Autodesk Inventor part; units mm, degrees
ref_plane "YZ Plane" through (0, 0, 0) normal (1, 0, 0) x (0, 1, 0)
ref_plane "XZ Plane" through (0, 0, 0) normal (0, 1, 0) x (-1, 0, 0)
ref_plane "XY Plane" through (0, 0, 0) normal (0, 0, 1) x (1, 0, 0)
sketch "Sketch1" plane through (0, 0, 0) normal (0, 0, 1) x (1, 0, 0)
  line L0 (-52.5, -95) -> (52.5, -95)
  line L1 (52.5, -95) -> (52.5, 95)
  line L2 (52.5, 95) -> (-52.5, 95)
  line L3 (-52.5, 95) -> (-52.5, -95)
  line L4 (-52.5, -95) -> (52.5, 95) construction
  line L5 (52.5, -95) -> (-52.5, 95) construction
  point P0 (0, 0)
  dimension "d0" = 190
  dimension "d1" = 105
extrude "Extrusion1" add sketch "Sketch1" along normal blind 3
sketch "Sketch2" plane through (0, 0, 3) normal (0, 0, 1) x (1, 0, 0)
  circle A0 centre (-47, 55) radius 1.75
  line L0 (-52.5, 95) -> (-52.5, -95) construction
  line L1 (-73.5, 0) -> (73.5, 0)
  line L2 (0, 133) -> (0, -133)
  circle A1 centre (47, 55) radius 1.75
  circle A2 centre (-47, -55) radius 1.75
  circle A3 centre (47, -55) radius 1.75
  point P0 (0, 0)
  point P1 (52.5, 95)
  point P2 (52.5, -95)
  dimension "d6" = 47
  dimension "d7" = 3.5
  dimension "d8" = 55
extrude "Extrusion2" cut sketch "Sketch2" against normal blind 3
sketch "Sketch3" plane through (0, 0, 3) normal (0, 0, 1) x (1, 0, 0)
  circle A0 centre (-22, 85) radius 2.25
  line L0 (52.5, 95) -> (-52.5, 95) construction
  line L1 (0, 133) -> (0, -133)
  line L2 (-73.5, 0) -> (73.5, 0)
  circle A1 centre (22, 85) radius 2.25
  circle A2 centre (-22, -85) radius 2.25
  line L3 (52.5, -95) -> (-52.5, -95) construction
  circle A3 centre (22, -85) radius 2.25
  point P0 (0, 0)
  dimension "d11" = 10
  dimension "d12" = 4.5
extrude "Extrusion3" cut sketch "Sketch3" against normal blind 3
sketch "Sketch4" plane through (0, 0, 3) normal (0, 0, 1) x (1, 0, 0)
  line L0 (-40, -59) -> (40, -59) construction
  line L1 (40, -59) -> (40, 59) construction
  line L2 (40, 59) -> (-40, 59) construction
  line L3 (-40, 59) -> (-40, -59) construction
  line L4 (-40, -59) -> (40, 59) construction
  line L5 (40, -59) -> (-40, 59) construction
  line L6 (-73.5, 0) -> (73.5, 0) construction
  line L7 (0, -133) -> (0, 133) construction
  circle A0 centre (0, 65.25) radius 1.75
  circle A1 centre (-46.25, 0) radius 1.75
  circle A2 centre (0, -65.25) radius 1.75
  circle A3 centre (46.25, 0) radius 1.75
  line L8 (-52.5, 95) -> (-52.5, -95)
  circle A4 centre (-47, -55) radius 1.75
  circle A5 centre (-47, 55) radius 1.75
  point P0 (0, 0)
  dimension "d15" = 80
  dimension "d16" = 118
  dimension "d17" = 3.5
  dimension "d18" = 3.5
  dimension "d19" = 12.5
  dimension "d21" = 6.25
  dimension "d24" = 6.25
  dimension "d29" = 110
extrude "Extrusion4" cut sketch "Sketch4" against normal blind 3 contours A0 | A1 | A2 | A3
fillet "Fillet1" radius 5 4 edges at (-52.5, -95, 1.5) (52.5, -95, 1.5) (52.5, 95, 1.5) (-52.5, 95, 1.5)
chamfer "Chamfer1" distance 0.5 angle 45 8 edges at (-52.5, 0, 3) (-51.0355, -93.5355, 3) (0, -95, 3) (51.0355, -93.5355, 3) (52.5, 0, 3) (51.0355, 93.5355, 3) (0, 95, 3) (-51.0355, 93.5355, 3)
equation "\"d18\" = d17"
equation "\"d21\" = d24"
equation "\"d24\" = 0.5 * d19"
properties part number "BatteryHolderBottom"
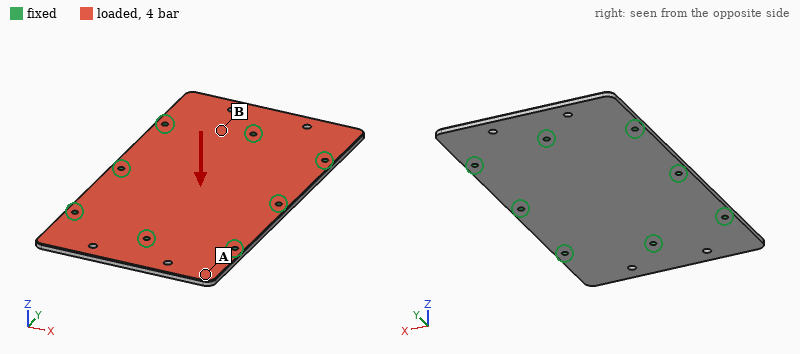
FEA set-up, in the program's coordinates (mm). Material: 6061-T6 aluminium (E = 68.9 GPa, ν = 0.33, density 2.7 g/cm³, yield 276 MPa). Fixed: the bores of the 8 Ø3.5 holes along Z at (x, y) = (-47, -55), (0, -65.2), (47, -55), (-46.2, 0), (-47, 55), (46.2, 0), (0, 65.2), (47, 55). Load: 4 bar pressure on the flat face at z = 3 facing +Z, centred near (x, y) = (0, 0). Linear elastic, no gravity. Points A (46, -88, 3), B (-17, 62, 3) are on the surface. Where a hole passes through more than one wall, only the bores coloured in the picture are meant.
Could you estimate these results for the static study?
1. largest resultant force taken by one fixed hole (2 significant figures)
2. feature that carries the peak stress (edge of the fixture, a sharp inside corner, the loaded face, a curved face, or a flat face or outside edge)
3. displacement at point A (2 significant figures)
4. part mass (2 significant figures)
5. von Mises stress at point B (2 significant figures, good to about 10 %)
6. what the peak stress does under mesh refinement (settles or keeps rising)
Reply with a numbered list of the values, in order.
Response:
1. 1.5 kN
2. edge of the fixture
3. 0.38 mm
4. 160 g
5. 94 MPa
6. keeps rising
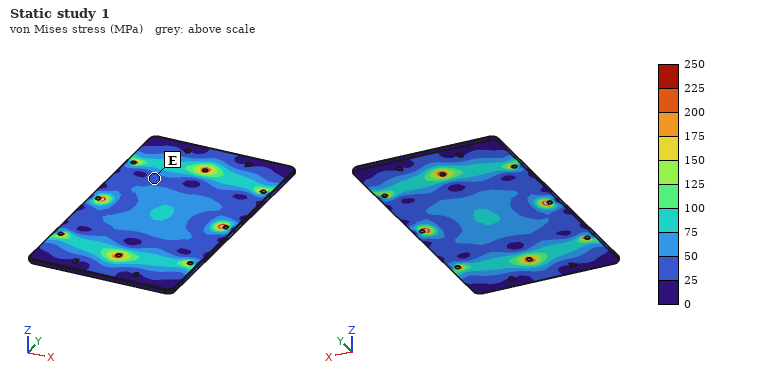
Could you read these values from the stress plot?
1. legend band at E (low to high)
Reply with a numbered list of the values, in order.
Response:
1. 25 to 50 MPa
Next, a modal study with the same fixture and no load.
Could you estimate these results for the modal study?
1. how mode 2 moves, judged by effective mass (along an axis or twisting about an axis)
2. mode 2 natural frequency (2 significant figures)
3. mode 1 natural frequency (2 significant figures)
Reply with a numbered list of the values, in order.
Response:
1. twisting about X
2. 1800 Hz
3. 1700 Hz
